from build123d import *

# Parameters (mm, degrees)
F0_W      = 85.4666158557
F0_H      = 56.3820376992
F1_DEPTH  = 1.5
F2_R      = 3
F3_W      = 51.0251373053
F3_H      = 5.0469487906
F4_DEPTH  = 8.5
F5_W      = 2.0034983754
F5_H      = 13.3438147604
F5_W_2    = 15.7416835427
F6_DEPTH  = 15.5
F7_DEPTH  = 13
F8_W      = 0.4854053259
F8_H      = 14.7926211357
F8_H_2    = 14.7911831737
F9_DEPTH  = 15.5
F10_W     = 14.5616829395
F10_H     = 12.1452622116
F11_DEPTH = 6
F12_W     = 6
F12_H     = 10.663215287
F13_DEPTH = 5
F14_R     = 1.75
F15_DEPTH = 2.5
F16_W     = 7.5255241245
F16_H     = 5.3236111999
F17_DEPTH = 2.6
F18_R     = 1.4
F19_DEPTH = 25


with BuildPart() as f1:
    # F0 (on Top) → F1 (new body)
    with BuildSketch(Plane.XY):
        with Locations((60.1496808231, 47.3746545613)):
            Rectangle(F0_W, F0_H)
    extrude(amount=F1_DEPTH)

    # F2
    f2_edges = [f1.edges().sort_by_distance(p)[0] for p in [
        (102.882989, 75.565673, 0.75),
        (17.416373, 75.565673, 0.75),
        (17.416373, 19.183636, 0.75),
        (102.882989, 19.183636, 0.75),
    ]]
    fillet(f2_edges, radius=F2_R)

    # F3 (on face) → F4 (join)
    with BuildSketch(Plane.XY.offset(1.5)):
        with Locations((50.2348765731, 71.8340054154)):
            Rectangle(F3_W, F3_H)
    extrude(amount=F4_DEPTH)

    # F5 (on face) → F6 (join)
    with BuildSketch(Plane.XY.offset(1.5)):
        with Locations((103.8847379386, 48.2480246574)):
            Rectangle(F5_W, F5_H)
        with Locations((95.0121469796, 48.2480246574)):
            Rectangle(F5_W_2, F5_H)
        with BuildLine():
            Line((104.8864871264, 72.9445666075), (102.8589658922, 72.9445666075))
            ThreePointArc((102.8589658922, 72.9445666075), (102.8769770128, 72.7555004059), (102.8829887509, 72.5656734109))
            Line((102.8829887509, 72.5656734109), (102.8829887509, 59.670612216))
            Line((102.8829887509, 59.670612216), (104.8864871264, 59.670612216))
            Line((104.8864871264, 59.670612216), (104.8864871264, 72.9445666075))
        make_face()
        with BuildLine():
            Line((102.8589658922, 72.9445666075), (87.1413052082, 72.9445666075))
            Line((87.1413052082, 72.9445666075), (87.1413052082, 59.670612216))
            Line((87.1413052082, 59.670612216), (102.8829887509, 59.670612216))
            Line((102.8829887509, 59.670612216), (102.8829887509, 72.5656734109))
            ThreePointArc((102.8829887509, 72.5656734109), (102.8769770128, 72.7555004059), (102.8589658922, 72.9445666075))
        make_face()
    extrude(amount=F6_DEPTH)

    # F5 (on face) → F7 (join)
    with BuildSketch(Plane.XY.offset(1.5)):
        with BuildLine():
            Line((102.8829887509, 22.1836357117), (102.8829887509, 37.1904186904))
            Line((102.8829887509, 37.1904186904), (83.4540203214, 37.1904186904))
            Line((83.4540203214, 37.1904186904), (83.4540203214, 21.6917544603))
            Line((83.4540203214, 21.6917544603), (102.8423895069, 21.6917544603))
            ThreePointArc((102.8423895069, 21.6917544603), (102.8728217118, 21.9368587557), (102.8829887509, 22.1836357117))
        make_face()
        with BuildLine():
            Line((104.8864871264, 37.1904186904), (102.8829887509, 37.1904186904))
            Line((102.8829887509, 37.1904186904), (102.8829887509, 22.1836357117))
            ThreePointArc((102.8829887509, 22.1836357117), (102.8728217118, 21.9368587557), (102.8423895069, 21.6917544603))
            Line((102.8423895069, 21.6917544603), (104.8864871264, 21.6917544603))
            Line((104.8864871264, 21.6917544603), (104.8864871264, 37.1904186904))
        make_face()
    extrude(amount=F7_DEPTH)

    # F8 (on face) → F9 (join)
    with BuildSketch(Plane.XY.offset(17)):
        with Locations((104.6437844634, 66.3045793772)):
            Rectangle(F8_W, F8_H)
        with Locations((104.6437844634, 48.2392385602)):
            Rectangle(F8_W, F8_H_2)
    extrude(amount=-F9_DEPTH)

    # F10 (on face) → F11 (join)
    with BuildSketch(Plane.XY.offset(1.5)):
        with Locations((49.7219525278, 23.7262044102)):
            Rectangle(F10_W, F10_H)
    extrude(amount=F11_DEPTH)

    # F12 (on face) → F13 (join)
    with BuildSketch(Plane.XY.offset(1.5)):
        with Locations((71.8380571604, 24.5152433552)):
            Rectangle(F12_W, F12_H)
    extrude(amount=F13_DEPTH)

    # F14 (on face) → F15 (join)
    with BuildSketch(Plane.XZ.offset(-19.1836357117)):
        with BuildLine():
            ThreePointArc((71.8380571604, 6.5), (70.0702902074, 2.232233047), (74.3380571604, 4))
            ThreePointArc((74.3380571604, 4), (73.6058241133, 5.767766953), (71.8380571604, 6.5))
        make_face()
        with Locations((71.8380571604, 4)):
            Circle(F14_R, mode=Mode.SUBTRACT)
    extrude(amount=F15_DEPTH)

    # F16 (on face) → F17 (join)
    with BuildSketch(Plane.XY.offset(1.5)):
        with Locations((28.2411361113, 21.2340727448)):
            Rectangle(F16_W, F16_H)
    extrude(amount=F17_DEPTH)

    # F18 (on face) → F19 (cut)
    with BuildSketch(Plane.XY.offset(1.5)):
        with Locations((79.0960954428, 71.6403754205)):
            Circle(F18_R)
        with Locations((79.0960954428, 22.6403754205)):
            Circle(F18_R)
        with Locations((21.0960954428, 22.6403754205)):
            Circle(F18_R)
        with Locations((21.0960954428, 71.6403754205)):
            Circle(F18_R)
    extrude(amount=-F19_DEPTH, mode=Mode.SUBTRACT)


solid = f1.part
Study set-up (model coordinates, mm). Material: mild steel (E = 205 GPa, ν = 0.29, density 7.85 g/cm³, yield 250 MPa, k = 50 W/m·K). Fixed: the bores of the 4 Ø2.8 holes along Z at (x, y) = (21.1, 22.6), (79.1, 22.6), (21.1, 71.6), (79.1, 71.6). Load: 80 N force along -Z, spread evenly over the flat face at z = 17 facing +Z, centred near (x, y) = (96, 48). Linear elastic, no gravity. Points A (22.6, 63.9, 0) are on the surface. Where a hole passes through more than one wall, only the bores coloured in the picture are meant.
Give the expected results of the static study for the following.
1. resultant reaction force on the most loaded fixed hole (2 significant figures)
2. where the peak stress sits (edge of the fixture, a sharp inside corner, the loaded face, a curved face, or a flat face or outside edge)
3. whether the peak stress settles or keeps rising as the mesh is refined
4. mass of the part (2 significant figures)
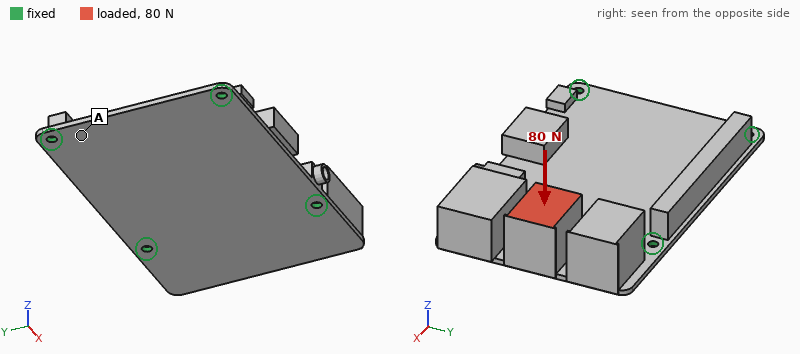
48 N
edge of the fixture
keeps rising
180 g
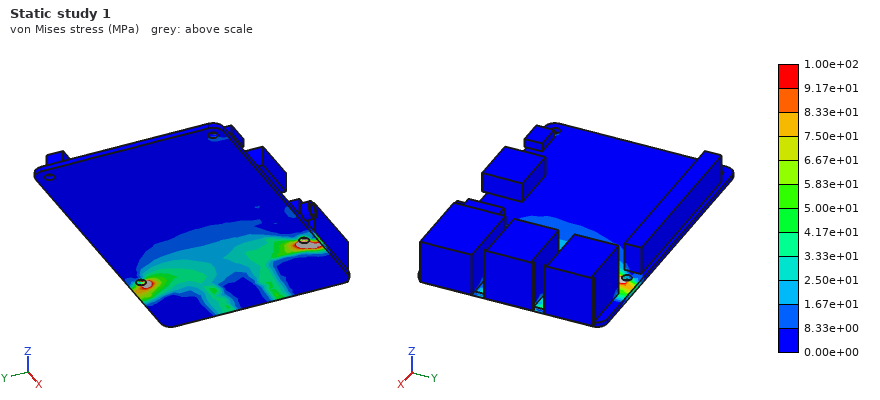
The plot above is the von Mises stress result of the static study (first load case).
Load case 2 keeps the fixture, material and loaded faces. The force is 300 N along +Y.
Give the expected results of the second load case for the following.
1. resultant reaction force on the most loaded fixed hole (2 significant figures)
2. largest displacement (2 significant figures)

220 N
77 µm
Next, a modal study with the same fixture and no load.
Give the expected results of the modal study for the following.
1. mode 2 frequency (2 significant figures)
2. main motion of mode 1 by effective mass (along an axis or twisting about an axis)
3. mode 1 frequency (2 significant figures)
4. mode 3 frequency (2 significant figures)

1700 Hz
along Z
530 Hz
1900 Hz
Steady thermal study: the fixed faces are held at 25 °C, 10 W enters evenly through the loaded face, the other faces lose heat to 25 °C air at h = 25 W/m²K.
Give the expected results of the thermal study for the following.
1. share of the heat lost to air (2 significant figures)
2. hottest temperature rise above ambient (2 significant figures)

46 %
52 K
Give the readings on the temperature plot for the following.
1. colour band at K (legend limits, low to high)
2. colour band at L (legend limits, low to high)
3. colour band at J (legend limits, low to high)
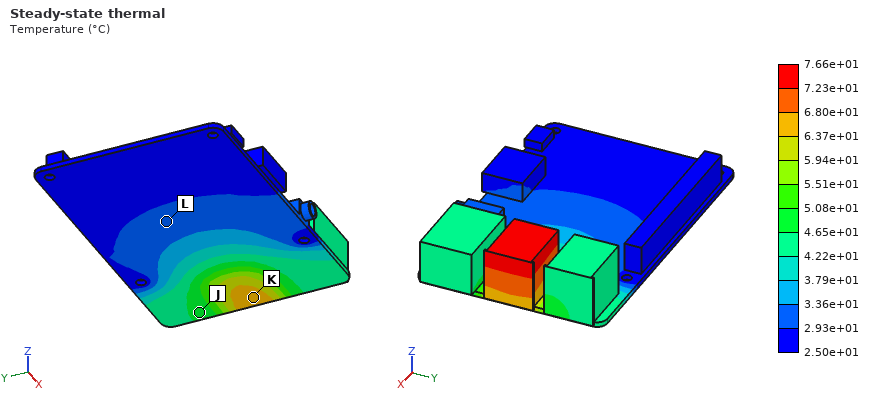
6.37e+01 to 6.80e+01 °C
2.93e+01 to 3.36e+01 °C
4.65e+01 to 5.08e+01 °C
